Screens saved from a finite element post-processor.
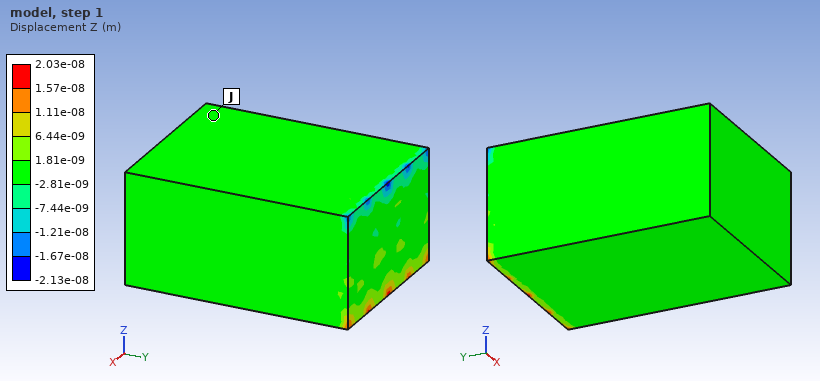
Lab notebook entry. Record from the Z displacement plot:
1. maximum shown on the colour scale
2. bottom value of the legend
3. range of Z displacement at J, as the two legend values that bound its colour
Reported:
2.03e-08 m
-2.13e-08 m
-2.81e-09 to 1.81e-09 m
